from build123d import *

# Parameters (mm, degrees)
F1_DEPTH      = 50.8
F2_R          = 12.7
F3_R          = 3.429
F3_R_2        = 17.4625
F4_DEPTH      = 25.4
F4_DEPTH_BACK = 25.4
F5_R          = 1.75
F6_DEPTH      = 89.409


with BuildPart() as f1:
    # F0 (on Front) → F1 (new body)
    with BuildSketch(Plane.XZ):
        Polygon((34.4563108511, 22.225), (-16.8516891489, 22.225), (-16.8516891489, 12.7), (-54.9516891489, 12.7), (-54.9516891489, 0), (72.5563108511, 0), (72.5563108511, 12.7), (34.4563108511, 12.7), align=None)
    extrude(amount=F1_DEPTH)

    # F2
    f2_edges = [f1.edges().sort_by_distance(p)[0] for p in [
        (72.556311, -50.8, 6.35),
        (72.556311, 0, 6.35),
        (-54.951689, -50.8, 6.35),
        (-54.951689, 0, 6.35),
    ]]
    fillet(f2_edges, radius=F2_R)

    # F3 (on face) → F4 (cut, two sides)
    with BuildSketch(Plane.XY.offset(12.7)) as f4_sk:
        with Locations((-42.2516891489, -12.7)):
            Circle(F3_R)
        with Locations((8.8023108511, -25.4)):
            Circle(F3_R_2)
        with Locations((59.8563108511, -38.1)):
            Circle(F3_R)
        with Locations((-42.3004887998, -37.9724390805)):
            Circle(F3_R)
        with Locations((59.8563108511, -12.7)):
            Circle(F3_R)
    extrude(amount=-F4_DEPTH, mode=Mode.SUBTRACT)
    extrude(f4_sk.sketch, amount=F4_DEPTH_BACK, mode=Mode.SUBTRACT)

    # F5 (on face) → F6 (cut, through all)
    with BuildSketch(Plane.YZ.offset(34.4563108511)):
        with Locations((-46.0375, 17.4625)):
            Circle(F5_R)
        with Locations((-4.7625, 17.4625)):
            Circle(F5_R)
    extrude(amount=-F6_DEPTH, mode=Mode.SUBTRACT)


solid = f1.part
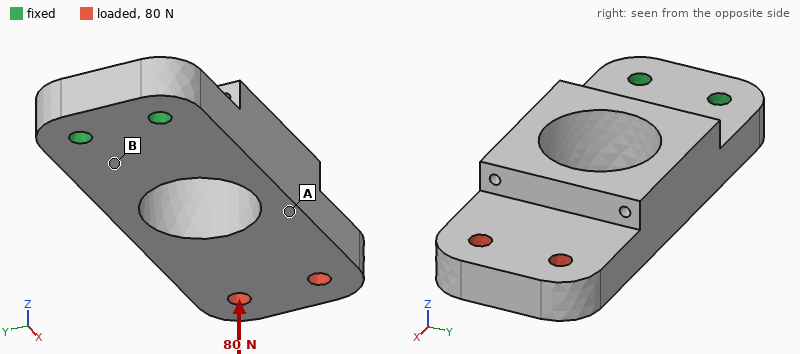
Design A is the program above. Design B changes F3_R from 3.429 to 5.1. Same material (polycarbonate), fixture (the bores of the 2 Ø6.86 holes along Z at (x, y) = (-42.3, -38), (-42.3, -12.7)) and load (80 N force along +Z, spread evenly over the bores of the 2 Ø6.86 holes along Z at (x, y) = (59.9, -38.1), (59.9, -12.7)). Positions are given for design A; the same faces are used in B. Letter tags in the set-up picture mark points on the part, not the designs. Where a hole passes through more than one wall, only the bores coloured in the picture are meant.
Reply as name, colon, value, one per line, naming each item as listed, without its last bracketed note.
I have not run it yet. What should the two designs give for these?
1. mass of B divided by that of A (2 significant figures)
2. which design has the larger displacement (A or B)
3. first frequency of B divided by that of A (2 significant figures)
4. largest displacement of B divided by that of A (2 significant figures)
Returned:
mass of B divided by that of A: 0.97
which design has the larger displacement: A
first frequency of B divided by that of A: 1.1
largest displacement of B divided by that of A: 0.92
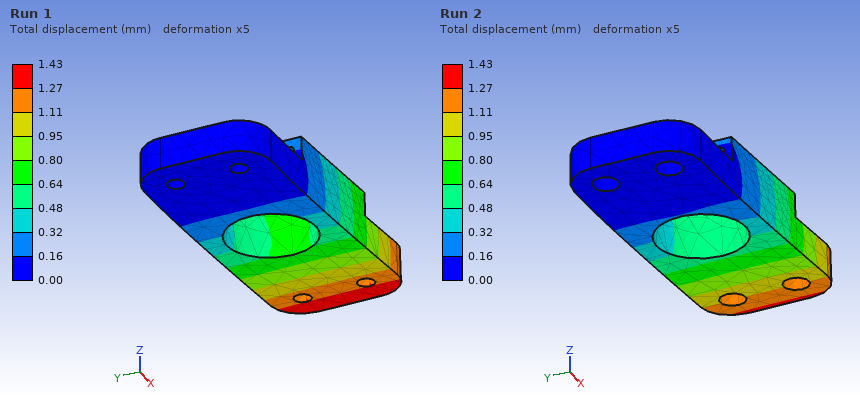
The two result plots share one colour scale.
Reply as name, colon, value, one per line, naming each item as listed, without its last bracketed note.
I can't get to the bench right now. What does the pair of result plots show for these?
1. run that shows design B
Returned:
run that shows design B: Run 2
